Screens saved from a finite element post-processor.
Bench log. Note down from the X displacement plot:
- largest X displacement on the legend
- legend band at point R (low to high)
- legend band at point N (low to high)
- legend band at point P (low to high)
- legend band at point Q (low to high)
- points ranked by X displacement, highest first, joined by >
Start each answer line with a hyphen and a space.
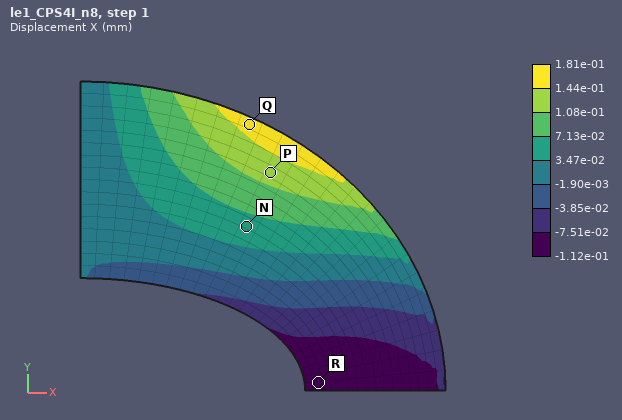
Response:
- 1.81e-01 mm
- -1.12e-01 to -7.51e-02 mm
- 3.47e-02 to 7.13e-02 mm
- 1.08e-01 to 1.44e-01 mm
- 1.44e-01 to 1.81e-01 mm
- Q > P > N > R
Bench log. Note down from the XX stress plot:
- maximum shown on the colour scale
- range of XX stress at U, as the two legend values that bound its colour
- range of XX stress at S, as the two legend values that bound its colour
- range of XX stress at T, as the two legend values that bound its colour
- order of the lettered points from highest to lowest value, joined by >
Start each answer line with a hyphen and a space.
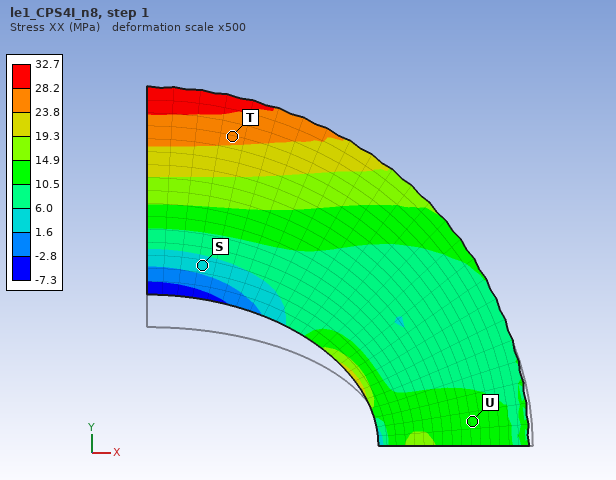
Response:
- 32.7 MPa
- 10.5 to 14.9 MPa
- 1.6 to 6.0 MPa
- 23.8 to 28.2 MPa
- T > U > S
